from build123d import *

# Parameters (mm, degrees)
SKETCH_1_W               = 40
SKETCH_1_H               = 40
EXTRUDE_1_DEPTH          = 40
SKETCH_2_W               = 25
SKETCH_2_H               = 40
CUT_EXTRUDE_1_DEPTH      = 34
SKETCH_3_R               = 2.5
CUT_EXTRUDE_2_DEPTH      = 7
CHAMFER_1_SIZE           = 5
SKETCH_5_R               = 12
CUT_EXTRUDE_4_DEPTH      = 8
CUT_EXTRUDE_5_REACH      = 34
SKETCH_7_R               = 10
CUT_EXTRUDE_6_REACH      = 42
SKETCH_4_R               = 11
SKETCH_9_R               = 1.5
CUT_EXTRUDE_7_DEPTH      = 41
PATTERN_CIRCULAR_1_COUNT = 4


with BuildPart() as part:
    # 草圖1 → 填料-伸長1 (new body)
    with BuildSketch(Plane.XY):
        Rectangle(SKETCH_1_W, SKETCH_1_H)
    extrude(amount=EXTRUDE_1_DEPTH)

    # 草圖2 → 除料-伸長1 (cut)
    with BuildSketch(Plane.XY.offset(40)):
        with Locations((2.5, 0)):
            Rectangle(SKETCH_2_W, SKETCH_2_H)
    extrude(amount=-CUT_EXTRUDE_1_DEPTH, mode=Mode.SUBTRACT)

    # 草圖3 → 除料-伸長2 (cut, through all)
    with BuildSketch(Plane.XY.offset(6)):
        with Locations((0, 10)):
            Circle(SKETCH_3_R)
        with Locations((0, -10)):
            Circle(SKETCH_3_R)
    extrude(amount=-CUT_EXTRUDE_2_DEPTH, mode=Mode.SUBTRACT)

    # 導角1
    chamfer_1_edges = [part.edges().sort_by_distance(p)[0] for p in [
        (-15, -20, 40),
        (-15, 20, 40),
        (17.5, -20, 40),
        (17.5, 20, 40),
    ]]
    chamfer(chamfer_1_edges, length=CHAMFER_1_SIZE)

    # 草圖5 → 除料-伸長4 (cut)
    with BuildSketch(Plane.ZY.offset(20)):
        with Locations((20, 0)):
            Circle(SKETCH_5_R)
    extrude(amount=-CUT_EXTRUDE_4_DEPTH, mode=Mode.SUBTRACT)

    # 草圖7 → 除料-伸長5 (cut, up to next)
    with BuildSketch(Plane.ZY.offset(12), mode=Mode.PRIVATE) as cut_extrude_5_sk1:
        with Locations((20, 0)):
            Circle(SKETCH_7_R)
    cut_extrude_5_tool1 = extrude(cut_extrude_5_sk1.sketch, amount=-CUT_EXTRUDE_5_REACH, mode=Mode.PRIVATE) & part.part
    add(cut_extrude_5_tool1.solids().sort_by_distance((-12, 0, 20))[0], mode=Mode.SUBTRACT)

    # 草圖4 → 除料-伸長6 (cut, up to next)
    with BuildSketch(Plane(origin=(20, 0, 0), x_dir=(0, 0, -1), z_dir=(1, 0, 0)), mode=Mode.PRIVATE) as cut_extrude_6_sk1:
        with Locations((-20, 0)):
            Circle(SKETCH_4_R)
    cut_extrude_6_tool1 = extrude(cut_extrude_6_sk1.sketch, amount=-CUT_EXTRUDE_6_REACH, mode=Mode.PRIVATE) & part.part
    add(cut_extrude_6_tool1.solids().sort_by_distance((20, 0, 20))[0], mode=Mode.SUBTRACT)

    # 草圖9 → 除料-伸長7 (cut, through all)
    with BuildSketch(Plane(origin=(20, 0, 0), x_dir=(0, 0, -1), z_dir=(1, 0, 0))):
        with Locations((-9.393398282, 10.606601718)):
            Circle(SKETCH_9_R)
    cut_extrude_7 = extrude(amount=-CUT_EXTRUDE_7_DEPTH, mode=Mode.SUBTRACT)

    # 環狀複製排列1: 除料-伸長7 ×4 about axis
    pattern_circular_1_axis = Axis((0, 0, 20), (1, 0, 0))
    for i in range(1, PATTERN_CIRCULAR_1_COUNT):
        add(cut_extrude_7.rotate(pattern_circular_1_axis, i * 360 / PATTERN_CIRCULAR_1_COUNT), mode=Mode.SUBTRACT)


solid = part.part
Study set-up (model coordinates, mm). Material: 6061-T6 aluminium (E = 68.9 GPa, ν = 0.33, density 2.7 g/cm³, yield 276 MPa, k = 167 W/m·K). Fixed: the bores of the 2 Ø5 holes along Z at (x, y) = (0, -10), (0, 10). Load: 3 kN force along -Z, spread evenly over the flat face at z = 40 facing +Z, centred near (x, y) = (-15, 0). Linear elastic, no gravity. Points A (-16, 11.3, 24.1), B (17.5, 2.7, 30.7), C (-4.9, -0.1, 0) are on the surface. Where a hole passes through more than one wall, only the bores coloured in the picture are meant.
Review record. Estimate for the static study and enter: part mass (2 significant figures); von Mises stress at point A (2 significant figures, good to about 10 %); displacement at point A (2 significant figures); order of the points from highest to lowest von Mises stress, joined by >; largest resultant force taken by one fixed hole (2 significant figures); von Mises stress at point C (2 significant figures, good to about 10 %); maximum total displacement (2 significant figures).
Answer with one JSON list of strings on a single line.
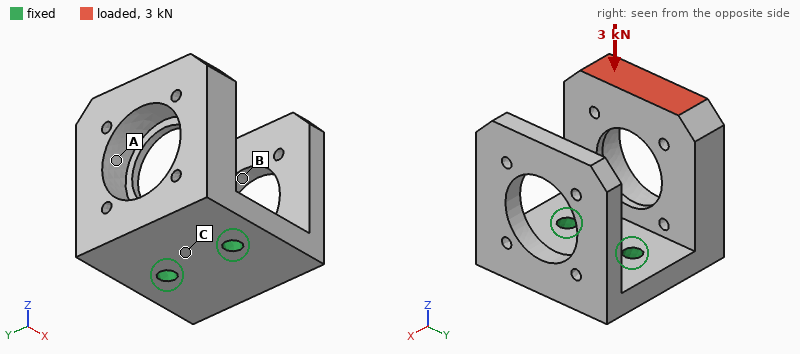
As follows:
["62 g", "54 MPa", "0.16 mm", "C > A > B", "1.5 kN", "78 MPa", "0.27 mm"]
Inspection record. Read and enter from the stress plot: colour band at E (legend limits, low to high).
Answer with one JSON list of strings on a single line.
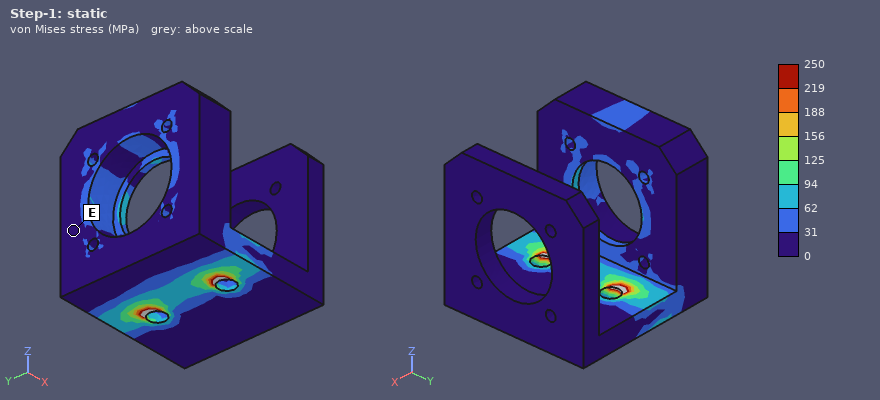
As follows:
["0 to 31 MPa"]
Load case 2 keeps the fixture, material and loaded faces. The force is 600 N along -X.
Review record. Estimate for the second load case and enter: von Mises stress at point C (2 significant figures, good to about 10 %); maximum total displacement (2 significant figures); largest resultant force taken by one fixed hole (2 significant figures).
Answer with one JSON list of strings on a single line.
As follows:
["64 MPa", "0.30 mm", "300 N"]
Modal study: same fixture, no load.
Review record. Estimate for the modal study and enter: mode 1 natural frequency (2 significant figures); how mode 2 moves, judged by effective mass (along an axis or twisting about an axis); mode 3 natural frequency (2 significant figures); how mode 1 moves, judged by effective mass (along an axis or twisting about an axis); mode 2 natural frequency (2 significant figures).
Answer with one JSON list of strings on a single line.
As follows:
["2000 Hz", "along X", "4100 Hz", "along X", "2300 Hz"]
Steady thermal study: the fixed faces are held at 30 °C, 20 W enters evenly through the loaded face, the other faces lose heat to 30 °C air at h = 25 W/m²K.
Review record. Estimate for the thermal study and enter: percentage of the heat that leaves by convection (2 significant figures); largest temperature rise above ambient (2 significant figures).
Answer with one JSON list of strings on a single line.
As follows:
["9.0 %", "27 K"]
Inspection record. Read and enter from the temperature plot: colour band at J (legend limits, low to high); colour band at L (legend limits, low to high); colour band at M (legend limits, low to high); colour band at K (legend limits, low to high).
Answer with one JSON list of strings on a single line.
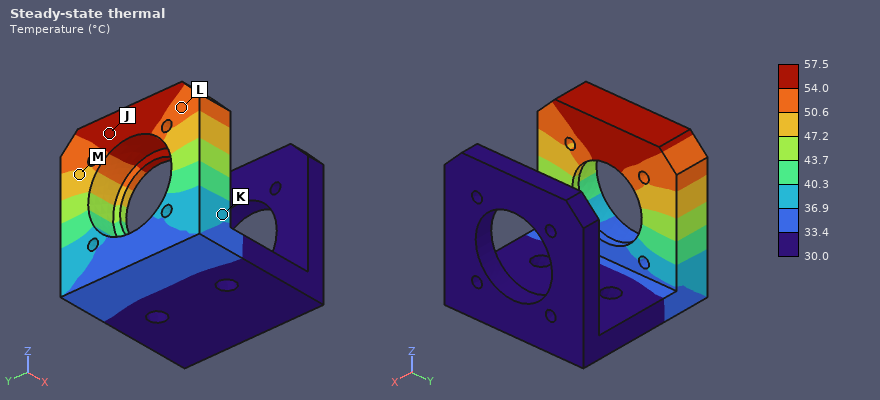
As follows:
["54.0 to 57.5 °C", "50.6 to 54.0 °C", "47.2 to 50.6 °C", "36.9 to 40.3 °C"]
